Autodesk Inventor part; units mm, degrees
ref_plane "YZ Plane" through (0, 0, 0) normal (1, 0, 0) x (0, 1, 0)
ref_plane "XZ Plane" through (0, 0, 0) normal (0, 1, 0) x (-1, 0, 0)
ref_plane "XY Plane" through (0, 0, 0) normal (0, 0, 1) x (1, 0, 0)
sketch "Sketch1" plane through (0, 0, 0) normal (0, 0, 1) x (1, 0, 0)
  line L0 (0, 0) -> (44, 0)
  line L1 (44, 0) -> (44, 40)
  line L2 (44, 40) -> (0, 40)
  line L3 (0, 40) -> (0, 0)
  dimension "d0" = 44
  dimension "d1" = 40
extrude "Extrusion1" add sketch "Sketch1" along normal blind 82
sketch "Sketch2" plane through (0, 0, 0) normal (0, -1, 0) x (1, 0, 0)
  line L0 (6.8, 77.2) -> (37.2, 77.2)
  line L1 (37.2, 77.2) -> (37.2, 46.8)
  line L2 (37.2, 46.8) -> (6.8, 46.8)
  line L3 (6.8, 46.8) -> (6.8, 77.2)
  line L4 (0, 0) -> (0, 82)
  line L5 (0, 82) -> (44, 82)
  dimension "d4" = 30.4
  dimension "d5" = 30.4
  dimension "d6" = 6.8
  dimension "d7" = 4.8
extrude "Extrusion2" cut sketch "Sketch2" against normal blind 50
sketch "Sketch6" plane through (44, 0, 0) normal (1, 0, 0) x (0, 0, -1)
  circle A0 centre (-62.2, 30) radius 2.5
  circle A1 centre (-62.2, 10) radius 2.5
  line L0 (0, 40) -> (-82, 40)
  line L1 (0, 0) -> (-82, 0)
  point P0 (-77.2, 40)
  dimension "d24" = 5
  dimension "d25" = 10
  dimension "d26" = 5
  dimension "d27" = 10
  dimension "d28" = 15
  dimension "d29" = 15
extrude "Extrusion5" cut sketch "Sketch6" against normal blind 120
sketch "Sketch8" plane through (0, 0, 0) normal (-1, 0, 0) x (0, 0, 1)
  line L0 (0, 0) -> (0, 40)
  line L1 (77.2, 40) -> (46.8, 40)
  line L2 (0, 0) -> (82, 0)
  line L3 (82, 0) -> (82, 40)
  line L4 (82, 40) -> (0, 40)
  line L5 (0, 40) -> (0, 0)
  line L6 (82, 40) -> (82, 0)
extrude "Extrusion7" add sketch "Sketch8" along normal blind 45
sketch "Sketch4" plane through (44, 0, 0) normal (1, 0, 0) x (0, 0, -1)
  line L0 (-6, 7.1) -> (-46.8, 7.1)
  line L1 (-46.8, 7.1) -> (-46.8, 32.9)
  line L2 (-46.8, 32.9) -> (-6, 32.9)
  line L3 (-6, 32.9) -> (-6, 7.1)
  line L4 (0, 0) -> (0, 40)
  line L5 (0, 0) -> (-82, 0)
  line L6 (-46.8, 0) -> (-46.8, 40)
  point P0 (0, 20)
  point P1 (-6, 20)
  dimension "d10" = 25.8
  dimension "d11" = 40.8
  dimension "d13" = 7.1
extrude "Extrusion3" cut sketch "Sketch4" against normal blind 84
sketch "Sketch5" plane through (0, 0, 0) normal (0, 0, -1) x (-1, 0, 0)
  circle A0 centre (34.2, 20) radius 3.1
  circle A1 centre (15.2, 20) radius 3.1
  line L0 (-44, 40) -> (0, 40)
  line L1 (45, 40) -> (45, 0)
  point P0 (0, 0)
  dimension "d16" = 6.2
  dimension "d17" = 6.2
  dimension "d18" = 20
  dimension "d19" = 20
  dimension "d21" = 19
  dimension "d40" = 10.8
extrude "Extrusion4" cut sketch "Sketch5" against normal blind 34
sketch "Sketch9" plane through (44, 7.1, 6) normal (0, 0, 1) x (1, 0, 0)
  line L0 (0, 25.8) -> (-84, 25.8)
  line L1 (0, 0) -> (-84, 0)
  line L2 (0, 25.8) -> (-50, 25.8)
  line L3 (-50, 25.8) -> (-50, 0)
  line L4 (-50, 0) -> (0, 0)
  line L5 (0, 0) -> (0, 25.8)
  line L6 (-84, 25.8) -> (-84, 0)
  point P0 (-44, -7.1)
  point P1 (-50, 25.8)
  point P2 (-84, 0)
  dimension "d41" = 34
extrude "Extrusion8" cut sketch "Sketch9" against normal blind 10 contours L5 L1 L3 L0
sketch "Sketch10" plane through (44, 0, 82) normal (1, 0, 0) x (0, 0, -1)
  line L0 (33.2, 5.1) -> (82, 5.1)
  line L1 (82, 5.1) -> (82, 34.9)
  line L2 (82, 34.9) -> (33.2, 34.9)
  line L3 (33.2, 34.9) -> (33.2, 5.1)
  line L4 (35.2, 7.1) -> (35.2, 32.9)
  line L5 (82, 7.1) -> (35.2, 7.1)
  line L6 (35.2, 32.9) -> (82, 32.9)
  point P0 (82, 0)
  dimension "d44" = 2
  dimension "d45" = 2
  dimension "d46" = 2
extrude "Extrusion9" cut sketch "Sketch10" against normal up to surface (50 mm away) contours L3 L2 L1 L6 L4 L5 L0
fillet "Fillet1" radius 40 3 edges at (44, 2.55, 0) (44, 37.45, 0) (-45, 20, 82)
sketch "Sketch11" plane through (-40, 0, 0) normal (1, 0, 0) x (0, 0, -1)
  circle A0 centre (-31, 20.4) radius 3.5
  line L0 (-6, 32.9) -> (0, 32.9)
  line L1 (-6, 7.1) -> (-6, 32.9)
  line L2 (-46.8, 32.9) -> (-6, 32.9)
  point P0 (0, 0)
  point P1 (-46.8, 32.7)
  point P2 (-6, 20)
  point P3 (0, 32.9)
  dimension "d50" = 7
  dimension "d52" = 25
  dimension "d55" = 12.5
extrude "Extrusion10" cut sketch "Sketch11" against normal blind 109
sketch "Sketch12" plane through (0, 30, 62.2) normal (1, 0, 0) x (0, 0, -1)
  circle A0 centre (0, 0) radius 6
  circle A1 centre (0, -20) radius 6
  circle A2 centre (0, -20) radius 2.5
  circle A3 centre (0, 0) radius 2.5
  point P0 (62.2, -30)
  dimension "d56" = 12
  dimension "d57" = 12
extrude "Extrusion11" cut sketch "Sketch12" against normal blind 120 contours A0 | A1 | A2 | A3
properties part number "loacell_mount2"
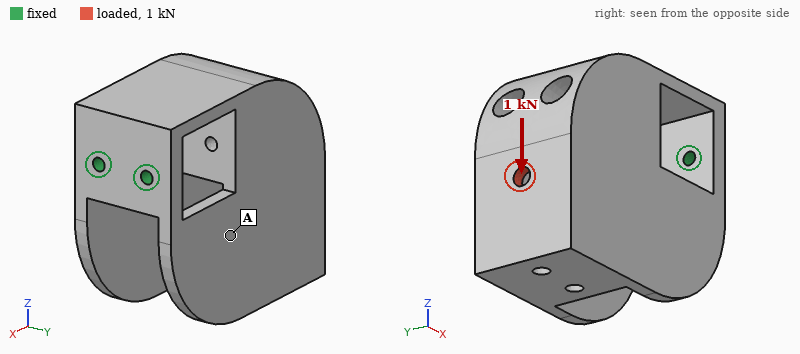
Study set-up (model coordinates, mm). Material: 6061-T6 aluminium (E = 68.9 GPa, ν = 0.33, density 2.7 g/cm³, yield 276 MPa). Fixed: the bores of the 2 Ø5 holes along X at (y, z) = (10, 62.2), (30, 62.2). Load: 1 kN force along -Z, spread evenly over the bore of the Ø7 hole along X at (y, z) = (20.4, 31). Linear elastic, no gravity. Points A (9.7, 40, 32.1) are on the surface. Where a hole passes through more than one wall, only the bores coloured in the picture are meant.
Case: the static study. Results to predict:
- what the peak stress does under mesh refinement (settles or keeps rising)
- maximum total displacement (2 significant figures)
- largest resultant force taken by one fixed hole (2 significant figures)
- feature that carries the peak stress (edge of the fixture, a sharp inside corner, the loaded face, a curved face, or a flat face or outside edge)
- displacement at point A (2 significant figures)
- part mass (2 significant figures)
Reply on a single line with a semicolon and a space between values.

keeps rising; 0.70 mm; 530 N; edge of the fixture; 0.30 mm; 330 g
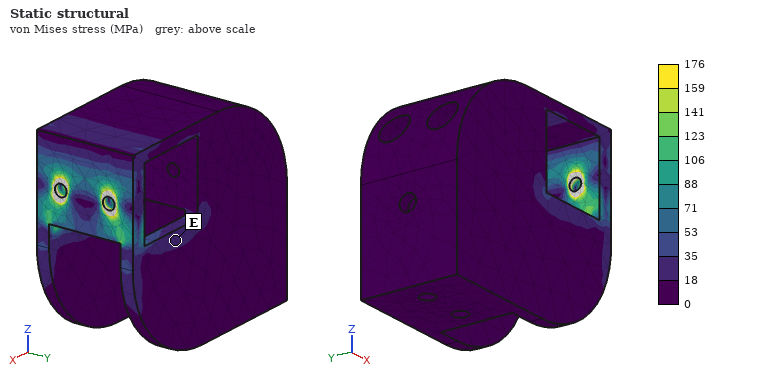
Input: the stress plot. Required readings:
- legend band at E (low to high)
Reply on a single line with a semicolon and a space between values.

18 to 35 MPa
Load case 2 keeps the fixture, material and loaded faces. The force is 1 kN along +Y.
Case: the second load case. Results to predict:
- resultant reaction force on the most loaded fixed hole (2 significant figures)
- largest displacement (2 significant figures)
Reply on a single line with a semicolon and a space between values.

3.3 kN; 0.49 mm
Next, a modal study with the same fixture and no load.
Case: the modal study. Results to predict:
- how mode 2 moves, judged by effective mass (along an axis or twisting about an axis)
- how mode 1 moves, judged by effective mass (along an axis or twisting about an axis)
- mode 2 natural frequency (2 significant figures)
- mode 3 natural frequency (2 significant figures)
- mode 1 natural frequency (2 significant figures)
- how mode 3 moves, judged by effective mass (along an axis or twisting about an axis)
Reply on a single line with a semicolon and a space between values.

along Y; along Z; 620 Hz; 1400 Hz; 500 Hz; twisting about X
